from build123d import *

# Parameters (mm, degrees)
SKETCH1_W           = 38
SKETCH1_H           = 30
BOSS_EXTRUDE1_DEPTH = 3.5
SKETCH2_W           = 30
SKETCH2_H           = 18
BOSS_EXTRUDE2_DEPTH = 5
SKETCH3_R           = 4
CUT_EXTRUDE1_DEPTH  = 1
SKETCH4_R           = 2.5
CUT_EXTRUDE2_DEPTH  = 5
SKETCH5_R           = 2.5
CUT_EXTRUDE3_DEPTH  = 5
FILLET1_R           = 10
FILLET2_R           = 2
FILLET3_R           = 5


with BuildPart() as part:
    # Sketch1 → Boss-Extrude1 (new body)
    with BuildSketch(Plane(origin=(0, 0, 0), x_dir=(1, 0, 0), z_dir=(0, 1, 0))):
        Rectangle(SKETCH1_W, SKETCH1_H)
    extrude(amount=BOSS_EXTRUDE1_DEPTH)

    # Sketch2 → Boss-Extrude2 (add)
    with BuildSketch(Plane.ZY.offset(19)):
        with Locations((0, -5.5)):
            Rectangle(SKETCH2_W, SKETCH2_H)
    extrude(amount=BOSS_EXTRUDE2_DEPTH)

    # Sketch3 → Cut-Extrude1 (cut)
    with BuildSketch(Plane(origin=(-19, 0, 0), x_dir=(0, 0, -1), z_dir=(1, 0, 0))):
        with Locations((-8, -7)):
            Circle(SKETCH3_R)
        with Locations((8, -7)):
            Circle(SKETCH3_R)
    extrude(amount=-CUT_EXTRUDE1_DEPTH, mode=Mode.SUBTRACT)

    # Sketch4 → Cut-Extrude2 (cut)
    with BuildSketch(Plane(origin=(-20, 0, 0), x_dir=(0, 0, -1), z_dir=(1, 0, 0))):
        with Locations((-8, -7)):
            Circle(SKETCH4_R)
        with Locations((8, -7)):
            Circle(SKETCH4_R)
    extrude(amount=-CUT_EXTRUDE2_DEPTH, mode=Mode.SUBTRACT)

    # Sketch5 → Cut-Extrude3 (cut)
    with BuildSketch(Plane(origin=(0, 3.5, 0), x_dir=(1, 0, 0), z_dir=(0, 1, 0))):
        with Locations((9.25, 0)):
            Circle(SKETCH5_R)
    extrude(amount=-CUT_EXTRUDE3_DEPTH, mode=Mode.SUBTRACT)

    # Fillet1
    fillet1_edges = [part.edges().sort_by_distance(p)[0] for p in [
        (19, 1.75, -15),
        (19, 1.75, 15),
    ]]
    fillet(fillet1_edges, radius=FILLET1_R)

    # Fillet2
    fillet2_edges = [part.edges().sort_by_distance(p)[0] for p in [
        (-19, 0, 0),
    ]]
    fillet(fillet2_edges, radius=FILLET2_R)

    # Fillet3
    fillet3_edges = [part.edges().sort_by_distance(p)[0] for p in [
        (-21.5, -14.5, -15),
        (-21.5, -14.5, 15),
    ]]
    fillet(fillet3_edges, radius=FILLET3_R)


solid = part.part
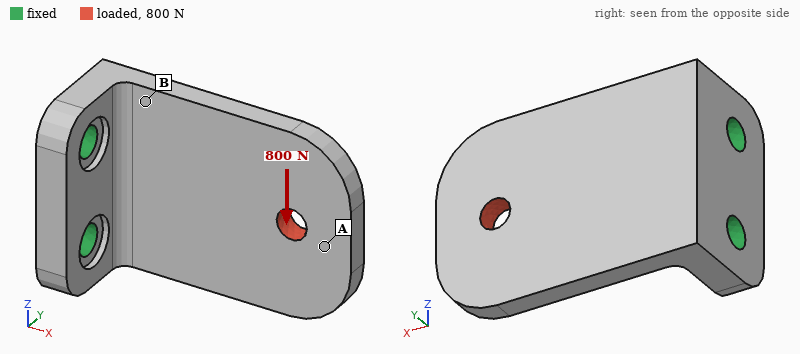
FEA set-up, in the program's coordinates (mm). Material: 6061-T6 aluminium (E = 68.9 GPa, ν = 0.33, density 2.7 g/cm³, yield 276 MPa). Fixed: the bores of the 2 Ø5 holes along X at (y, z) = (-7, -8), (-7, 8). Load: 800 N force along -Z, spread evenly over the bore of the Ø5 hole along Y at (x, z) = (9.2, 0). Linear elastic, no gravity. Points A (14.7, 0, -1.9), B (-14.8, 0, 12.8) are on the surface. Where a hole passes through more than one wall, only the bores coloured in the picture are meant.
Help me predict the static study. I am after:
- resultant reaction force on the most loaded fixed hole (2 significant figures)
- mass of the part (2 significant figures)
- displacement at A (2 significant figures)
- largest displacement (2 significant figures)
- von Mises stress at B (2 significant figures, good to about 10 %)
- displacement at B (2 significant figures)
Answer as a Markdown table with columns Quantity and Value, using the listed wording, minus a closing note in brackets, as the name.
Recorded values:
| Quantity | Value |
|---|---|
| resultant reaction force on the most loaded fixed hole | 1.4 kN |
| mass of the part | 17 g |
| displacement at A | 0.11 mm |
| largest displacement | 0.13 mm |
| von Mises stress at B | 66 MPa |
| displacement at B | 0.039 mm |
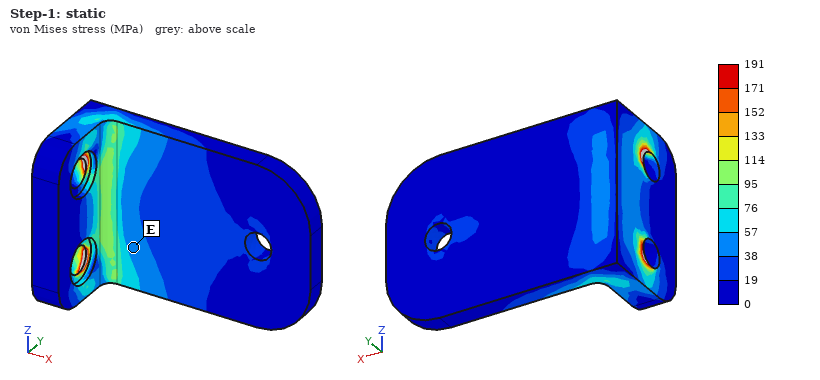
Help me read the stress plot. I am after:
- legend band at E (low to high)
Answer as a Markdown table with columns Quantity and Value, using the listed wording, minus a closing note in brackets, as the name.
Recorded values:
| Quantity | Value |
|---|---|
| legend band at E | 38 to 57 MPa |
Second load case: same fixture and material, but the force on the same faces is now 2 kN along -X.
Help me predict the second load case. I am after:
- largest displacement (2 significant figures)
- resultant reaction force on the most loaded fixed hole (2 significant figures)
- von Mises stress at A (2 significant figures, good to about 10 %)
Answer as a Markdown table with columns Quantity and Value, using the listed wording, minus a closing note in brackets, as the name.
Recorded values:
| Quantity | Value |
|---|---|
| largest displacement | 0.17 mm |
| resultant reaction force on the most loaded fixed hole | 1.0 kN |
| von Mises stress at A | 24 MPa |
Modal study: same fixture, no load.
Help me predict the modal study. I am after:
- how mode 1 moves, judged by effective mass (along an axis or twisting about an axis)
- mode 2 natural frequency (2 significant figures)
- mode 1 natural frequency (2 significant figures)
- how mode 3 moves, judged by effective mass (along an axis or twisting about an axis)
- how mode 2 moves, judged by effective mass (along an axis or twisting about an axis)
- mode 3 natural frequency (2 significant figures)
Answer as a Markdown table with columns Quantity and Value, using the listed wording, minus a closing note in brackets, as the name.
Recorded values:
| Quantity | Value |
|---|---|
| how mode 1 moves, judged by effective mass | along Y |
| mode 2 natural frequency | 5200 Hz |
| mode 1 natural frequency | 1800 Hz |
| how mode 3 moves, judged by effective mass | along Z |
| how mode 2 moves, judged by effective mass | along Z |
| mode 3 natural frequency | 6700 Hz |
